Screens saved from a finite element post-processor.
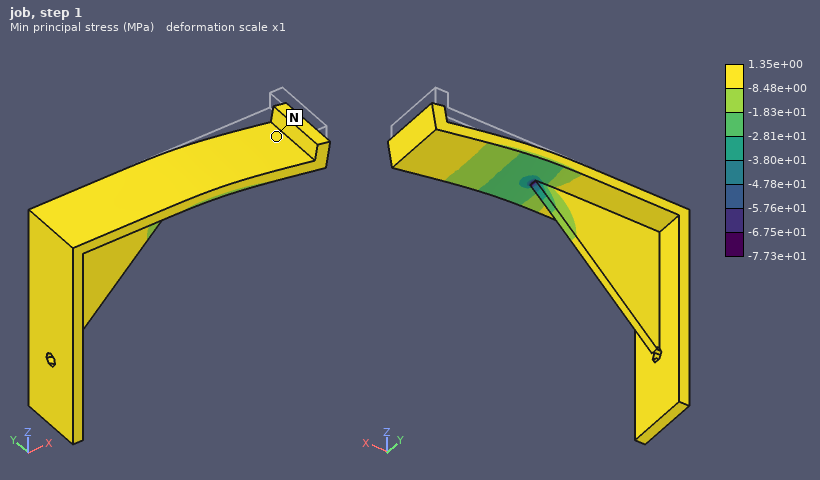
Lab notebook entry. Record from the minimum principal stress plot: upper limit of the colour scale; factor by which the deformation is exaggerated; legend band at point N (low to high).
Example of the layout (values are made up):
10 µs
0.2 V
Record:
1.35e+00 MPa
1
-8.48e+00 to 1.35e+00 MPa
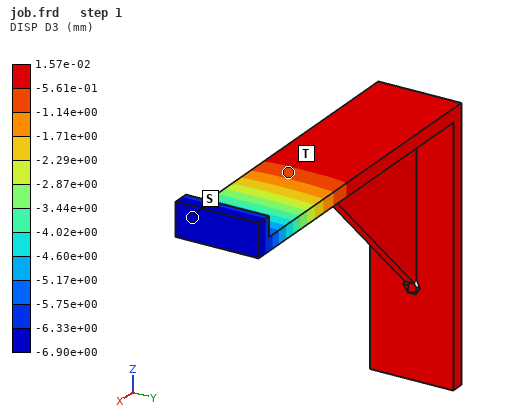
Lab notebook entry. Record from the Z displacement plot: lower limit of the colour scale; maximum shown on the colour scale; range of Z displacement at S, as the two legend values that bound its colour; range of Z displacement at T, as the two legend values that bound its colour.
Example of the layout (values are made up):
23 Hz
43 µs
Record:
-6.90e+00 mm
1.57e-02 mm
-6.90e+00 to -6.33e+00 mm
-1.14e+00 to -5.61e-01 mm
